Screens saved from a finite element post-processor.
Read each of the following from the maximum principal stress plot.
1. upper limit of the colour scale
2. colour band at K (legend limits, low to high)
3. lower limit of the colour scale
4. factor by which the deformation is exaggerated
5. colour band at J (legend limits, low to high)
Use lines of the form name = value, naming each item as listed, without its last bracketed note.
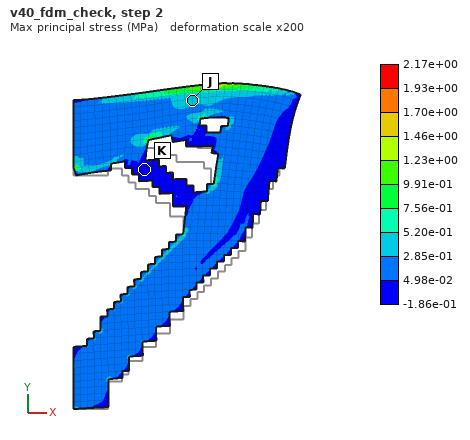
upper limit of the colour scale = 2.17e+00 MPa
colour band at K = -1.86e-01 to 4.98e-02 MPa
lower limit of the colour scale = -1.86e-01 MPa
factor by which the deformation is exaggerated = 200
colour band at J = 2.85e-01 to 5.20e-01 MPa
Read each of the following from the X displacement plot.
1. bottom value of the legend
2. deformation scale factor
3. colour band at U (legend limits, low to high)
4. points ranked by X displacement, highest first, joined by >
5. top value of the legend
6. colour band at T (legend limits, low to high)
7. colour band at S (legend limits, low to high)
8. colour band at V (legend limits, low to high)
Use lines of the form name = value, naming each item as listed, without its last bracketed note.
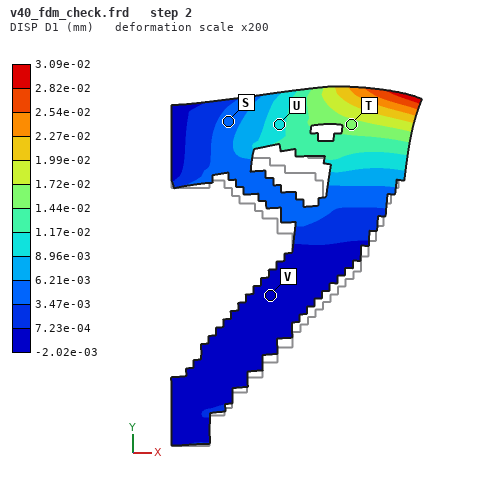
bottom value of the legend = -2.02e-03 mm
deformation scale factor = 200
colour band at U = 8.96e-03 to 1.17e-02 mm
points ranked by X displacement, highest first, joined by > = T > U > S > V
top value of the legend = 3.09e-02 mm
colour band at T = 1.44e-02 to 1.72e-02 mm
colour band at S = 3.47e-03 to 6.21e-03 mm
colour band at V = -2.02e-03 to 7.23e-04 mm
